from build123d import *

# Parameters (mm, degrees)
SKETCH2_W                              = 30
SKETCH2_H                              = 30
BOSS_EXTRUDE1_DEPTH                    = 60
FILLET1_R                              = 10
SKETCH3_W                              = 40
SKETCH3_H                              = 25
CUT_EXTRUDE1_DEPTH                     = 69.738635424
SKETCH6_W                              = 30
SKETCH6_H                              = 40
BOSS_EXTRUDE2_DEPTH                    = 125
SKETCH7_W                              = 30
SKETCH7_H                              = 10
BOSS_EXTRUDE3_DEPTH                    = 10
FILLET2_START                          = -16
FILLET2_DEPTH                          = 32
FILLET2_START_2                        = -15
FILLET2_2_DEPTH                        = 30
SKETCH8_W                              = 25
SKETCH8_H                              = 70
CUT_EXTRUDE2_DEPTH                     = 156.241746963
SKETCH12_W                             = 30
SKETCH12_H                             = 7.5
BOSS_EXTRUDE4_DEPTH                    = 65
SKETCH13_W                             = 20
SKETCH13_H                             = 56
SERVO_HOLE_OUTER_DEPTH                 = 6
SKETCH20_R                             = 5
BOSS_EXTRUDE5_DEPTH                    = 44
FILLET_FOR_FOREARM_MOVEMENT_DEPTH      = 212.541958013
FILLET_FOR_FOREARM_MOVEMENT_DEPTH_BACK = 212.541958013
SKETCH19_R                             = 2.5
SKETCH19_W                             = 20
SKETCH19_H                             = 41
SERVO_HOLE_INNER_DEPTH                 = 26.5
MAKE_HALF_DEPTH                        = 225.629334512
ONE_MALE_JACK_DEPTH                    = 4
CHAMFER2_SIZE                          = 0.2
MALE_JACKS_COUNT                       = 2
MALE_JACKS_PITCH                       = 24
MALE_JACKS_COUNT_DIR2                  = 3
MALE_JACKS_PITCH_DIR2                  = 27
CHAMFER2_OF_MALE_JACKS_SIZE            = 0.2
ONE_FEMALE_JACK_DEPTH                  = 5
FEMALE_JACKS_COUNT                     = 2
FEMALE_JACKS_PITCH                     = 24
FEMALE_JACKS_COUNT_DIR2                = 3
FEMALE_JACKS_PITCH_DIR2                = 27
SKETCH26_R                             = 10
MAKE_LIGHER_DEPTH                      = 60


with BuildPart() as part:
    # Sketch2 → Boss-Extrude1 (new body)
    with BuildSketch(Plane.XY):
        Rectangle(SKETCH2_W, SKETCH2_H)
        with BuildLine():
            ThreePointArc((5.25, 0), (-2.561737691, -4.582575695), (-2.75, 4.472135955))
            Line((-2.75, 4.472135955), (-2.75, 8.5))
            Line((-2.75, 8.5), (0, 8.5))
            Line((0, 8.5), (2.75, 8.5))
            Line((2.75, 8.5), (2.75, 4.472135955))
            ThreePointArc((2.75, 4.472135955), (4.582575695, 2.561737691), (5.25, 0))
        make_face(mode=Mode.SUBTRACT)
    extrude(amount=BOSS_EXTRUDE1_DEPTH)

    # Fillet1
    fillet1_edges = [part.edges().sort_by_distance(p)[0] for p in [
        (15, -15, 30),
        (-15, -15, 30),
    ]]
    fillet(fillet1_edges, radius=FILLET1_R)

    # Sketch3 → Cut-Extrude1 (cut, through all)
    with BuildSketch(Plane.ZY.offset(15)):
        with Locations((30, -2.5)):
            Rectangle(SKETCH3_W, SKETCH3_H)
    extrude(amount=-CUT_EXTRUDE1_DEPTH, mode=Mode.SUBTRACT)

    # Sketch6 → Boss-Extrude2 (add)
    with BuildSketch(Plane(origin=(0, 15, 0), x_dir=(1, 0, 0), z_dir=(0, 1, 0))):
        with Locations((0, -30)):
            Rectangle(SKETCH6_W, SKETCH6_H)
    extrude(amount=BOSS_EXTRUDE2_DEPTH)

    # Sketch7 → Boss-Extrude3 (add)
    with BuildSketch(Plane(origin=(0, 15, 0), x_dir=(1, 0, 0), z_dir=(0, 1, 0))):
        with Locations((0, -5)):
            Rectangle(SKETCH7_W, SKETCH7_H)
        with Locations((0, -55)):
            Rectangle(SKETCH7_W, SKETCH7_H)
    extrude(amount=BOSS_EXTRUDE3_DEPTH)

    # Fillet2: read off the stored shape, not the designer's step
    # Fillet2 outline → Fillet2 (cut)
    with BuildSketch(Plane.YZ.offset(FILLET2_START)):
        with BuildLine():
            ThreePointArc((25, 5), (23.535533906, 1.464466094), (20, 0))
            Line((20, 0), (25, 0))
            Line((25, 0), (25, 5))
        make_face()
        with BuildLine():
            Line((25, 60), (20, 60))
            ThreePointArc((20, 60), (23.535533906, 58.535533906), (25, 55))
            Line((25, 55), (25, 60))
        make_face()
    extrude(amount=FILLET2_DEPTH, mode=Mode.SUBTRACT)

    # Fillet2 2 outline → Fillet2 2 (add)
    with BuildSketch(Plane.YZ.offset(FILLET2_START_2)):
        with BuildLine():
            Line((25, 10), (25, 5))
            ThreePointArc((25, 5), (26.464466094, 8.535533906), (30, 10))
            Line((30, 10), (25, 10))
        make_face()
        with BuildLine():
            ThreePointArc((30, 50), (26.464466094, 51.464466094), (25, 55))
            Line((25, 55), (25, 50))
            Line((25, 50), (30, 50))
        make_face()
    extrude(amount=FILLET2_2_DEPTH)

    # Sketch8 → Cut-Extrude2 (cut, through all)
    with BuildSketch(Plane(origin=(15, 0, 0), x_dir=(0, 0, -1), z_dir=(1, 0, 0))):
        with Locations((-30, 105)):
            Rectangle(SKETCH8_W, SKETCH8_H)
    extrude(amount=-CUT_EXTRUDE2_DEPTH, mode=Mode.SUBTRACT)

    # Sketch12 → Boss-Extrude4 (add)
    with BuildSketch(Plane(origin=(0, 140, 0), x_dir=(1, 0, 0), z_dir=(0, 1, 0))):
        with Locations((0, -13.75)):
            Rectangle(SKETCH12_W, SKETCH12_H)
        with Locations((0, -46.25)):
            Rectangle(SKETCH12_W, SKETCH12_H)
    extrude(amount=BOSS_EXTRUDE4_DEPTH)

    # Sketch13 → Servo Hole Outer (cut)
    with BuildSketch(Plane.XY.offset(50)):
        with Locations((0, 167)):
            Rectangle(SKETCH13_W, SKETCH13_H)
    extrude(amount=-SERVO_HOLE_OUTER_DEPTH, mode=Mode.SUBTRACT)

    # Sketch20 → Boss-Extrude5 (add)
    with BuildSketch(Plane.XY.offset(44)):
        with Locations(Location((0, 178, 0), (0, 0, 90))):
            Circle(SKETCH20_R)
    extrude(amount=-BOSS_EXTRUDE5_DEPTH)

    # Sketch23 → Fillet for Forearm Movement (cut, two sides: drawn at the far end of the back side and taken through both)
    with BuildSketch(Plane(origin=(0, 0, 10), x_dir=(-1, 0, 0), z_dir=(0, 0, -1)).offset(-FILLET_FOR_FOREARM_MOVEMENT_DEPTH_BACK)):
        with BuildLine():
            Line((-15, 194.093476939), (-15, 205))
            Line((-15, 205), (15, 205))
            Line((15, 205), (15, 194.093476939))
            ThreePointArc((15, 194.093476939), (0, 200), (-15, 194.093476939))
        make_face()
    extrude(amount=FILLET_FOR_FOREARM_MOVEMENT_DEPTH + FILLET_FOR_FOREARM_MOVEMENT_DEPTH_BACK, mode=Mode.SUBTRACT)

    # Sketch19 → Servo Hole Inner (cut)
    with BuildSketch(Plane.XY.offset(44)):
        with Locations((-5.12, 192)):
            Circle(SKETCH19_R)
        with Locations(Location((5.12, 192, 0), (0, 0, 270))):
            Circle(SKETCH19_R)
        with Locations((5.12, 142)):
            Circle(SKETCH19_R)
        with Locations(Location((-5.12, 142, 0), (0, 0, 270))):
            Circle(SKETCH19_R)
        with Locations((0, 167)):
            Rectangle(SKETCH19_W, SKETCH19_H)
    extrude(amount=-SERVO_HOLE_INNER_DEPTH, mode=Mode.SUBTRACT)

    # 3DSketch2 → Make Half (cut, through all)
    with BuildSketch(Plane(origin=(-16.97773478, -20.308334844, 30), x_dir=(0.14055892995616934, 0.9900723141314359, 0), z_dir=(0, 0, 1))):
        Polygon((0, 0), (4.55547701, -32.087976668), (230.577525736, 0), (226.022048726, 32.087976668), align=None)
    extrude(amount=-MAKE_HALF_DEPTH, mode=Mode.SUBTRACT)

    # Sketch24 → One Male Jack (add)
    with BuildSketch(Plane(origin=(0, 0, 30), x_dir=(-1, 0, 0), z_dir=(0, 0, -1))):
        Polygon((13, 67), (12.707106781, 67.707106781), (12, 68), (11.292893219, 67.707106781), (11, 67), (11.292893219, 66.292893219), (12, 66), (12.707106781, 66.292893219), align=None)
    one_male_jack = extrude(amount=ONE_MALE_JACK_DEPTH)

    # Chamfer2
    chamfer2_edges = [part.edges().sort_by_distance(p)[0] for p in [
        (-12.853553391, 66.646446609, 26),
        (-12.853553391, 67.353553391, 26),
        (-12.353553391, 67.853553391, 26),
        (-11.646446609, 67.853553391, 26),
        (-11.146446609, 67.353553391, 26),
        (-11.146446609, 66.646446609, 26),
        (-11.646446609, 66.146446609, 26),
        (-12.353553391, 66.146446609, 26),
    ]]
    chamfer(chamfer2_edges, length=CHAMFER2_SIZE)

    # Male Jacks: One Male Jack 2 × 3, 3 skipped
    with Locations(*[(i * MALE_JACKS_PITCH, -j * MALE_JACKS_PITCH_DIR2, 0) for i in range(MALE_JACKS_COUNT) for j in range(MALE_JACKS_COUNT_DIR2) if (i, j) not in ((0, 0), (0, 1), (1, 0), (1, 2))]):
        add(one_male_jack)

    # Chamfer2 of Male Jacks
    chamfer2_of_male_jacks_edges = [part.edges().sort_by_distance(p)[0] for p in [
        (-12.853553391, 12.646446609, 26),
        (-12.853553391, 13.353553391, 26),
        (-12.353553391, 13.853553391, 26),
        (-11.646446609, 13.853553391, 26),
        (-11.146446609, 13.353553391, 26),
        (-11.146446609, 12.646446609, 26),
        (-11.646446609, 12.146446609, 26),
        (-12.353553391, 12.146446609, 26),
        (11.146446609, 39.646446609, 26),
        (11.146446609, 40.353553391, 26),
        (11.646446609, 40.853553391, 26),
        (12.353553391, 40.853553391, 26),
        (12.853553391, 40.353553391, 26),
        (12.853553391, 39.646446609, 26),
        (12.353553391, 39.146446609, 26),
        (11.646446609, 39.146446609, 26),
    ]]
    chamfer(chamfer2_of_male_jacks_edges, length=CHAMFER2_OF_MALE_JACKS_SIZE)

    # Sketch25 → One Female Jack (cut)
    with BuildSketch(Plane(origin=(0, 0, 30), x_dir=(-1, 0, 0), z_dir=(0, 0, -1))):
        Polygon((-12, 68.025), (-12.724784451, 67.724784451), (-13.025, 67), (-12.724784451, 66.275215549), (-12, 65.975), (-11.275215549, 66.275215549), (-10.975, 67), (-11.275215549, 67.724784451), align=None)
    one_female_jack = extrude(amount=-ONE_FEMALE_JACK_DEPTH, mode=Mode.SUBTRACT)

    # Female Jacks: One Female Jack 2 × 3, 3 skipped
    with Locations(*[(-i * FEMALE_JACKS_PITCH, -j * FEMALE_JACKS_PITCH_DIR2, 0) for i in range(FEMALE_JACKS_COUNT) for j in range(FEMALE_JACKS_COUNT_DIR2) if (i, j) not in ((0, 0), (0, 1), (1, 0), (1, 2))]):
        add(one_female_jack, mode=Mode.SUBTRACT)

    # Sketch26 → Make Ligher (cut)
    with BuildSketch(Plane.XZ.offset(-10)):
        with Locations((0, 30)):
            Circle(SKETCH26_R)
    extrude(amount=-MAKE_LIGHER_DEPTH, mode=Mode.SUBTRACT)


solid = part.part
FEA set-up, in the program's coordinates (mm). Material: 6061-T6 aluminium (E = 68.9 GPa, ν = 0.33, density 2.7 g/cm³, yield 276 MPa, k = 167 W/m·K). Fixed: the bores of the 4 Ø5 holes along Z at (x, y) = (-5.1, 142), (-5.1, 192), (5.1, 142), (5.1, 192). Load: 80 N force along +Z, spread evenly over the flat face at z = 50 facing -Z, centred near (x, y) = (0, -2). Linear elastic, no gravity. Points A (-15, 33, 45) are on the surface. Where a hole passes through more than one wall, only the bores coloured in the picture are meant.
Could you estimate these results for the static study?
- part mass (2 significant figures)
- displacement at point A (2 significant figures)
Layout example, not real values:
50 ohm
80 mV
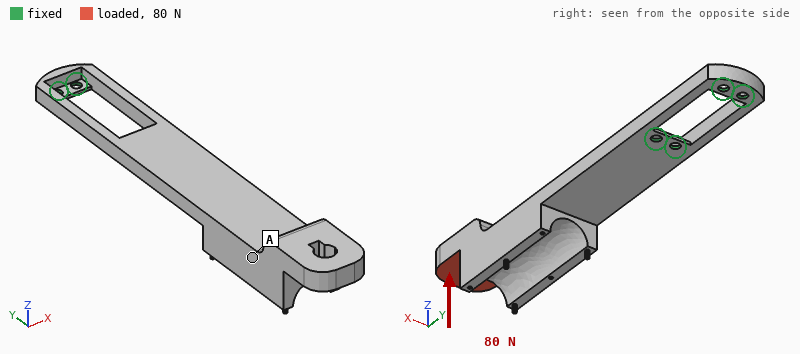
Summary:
160 g
1.2 mm
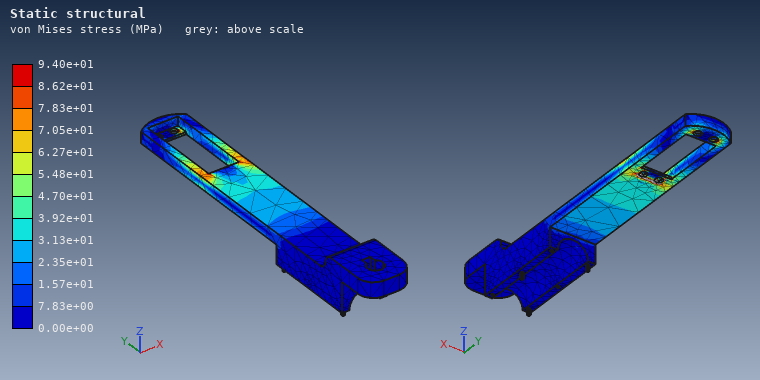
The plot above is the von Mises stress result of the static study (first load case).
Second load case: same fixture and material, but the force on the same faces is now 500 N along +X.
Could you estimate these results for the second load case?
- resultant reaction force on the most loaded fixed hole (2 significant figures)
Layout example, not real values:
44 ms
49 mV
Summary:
3.5 kN
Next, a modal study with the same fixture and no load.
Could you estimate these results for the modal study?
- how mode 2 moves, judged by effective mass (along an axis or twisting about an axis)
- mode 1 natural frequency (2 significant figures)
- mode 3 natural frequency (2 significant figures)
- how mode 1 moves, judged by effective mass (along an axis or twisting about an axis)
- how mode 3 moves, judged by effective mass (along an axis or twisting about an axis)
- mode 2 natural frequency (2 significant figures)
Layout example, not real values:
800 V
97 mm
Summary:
along X
140 Hz
1300 Hz
along Z
twisting about Y
530 Hz
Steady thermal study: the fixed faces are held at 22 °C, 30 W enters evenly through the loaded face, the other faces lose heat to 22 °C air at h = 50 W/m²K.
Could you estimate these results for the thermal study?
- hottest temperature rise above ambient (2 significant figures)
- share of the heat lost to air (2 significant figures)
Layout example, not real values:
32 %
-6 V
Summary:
51 K
68 %
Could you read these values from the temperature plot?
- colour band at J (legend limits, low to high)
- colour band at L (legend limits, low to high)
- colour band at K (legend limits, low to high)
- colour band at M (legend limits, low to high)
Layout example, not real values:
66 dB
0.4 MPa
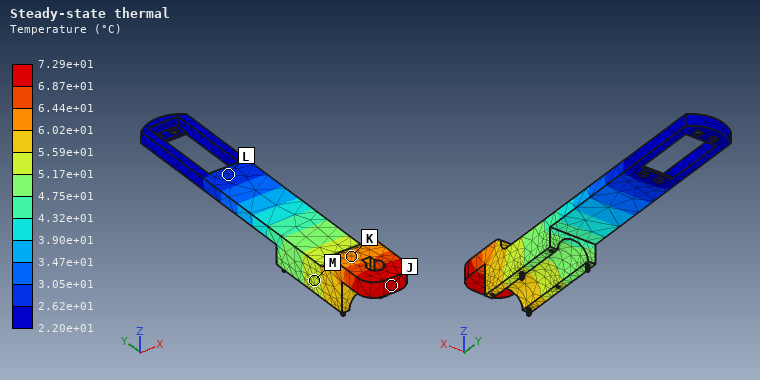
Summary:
6.87e+01 to 7.29e+01 °C
2.62e+01 to 3.05e+01 °C
6.02e+01 to 6.44e+01 °C
5.17e+01 to 5.59e+01 °C
